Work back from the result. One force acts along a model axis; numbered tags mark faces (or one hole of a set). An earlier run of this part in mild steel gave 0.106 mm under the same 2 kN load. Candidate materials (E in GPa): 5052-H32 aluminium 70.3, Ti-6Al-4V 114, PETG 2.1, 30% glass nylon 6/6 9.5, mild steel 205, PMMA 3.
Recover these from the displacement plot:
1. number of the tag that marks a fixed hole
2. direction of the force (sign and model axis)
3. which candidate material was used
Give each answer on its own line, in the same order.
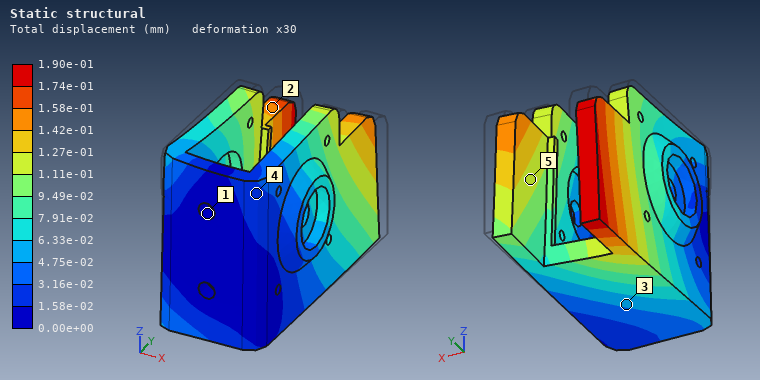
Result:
1
-Z
Ti-6Al-4V
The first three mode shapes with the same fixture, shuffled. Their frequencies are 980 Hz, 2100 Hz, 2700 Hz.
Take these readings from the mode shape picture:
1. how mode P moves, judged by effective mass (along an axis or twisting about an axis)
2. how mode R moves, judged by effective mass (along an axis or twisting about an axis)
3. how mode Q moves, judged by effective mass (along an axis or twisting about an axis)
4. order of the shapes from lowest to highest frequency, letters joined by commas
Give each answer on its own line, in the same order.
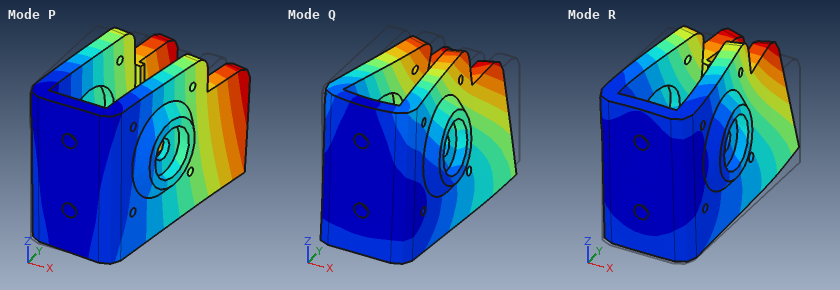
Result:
along X
along Z
along Z
P, Q, R
